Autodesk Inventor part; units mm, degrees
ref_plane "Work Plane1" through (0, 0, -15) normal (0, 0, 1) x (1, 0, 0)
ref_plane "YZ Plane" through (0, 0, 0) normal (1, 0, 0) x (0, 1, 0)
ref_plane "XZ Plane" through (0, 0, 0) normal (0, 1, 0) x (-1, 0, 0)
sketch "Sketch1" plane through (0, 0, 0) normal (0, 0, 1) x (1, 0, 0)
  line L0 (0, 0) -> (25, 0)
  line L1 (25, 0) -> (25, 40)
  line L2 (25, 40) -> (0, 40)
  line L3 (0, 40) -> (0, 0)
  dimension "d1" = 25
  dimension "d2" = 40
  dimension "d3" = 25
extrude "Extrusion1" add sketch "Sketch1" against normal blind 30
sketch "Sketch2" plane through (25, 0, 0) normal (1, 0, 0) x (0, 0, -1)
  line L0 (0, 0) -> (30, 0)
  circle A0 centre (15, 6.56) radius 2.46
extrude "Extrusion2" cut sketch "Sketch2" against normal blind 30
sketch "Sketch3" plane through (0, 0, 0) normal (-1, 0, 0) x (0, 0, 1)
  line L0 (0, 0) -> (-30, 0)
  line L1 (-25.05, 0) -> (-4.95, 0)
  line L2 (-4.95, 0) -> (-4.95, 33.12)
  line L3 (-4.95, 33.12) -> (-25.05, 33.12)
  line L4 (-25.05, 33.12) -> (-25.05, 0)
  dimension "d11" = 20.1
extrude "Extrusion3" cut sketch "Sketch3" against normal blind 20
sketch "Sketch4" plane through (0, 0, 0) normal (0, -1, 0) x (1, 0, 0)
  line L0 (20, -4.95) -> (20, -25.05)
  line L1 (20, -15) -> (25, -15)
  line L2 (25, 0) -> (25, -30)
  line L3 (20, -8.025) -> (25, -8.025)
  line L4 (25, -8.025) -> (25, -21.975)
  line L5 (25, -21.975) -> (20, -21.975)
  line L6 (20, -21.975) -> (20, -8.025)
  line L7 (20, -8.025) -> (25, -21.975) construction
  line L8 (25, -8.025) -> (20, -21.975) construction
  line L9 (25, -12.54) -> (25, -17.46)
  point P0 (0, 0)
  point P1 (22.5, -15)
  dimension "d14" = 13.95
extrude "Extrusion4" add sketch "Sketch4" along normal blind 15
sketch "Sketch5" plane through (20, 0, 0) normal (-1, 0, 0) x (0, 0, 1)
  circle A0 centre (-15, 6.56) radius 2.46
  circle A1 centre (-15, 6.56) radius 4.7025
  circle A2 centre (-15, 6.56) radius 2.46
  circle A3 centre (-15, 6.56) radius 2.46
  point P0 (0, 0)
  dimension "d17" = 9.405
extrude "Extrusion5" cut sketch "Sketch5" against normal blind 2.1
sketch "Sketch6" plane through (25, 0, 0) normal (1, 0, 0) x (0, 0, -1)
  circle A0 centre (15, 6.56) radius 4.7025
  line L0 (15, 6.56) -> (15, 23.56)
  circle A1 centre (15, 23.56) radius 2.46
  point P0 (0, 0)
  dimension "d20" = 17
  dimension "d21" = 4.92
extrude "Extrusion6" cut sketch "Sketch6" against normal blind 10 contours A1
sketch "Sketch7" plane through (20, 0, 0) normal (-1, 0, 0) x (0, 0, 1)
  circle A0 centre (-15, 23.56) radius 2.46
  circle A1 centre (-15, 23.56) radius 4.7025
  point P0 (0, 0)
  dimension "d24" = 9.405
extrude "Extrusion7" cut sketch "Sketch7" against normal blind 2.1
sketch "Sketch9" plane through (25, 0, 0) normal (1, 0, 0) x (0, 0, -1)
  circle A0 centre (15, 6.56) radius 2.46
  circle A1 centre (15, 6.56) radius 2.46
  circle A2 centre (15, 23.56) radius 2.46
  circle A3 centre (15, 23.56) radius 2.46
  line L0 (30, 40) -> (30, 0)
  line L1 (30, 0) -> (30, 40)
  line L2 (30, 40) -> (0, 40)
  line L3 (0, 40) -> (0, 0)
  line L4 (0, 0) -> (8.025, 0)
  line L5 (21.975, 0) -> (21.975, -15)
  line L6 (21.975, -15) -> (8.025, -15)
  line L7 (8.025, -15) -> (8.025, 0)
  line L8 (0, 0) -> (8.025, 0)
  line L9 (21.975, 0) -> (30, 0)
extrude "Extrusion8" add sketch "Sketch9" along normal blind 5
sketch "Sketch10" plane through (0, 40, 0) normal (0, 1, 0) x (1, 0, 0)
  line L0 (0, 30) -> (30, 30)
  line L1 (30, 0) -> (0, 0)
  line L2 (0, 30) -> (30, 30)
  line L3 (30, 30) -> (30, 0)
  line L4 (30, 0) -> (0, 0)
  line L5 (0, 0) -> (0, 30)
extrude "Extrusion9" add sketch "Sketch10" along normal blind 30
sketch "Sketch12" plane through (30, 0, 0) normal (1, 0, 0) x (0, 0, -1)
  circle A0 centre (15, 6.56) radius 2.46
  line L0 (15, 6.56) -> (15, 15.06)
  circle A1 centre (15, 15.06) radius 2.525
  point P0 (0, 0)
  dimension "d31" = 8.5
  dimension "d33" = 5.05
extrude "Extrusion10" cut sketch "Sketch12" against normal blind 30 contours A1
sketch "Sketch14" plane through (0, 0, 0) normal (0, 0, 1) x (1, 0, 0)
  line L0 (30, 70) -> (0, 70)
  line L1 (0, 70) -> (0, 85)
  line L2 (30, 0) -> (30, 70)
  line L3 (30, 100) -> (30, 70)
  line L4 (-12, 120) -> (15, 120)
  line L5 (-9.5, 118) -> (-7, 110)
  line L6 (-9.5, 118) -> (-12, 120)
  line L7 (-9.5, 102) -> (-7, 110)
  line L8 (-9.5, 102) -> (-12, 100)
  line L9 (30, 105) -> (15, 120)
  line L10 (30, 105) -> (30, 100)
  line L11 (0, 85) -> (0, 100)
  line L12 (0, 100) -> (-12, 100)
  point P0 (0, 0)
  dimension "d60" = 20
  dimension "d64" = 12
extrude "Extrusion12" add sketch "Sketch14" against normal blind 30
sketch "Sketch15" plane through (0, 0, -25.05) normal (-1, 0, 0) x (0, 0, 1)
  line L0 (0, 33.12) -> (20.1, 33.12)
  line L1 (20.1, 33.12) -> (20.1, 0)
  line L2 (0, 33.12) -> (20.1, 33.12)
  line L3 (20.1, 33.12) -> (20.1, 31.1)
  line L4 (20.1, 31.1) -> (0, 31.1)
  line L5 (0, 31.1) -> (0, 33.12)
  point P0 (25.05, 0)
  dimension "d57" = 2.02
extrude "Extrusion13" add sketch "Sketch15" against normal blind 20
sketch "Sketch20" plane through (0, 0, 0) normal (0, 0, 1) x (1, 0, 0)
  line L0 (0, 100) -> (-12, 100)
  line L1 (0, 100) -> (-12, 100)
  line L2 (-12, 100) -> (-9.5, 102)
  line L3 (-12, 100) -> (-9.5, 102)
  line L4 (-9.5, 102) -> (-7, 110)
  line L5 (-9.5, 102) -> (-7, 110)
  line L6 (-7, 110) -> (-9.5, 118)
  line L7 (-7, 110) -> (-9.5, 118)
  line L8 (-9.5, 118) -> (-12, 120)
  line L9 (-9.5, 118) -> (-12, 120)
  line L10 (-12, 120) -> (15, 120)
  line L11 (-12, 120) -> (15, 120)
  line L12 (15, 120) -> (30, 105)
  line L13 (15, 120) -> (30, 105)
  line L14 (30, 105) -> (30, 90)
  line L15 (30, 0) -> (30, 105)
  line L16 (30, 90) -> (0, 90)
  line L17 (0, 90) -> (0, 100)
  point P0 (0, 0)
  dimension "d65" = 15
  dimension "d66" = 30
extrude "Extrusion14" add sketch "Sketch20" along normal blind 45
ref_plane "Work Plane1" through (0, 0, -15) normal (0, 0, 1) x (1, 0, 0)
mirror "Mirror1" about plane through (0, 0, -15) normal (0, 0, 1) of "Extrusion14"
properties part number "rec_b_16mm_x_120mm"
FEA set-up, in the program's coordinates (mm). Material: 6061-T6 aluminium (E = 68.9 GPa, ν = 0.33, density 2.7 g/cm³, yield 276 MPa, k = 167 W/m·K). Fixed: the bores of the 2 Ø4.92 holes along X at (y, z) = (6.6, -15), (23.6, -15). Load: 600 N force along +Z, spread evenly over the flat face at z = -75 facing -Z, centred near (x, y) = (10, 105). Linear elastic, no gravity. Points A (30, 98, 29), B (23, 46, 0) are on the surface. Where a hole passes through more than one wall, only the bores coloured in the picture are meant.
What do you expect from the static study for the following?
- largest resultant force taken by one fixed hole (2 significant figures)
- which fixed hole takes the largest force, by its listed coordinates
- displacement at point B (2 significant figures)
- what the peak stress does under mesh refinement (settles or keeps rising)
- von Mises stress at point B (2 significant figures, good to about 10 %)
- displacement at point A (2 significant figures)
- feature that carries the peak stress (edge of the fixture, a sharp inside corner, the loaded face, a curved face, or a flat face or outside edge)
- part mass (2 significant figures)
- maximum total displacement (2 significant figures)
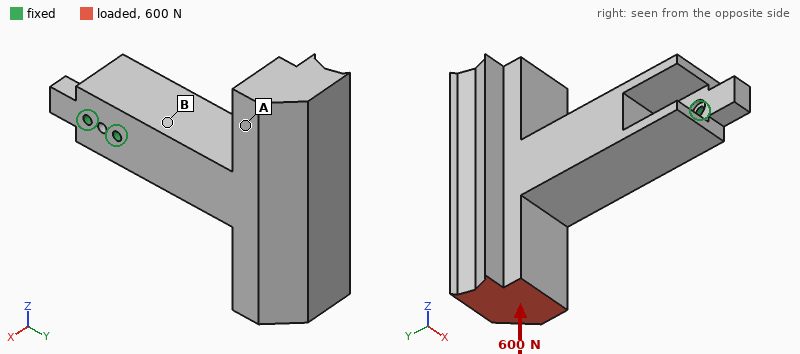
2.7 kN
(23.6, -15)
0.022 mm
keeps rising
9.3 MPa
0.083 mm
edge of the fixture
500 g
0.12 mm
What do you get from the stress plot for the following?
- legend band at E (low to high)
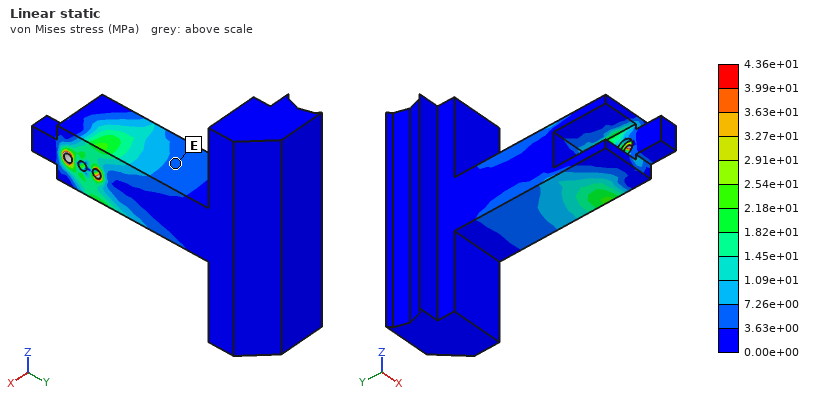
3.63e+00 to 7.26e+00 MPa
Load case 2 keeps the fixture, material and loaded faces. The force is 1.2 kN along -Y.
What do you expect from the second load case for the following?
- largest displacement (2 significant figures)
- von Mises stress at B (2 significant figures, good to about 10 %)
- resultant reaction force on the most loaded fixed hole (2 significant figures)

0.24 mm
20 MPa
3.3 kN
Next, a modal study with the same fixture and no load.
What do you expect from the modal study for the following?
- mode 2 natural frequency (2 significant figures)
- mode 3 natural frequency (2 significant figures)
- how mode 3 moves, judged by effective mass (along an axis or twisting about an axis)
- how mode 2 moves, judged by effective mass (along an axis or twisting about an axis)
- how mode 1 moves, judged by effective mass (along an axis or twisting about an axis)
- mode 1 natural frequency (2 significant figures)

670 Hz
930 Hz
twisting about Y
along Z
along X
620 Hz
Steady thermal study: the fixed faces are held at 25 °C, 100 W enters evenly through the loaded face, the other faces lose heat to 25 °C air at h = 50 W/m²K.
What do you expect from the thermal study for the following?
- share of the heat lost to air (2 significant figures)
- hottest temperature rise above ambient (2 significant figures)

47 %
69 K
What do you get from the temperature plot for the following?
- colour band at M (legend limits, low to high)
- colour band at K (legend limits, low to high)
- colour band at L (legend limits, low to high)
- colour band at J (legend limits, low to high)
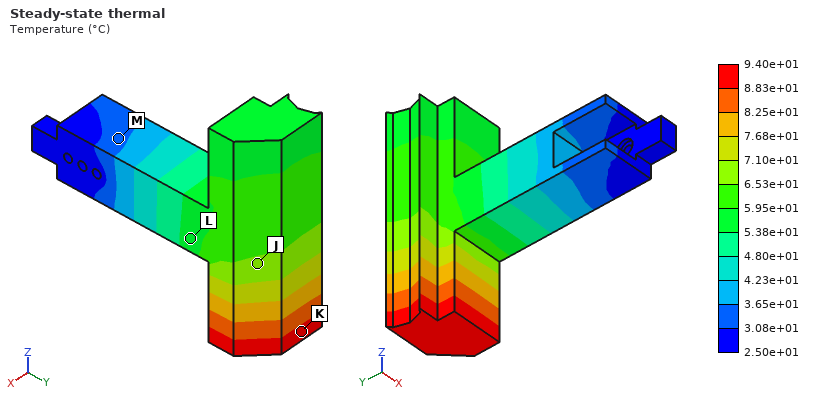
3.08e+01 to 3.65e+01 °C
8.83e+01 to 9.40e+01 °C
5.38e+01 to 5.95e+01 °C
6.53e+01 to 7.10e+01 °C
